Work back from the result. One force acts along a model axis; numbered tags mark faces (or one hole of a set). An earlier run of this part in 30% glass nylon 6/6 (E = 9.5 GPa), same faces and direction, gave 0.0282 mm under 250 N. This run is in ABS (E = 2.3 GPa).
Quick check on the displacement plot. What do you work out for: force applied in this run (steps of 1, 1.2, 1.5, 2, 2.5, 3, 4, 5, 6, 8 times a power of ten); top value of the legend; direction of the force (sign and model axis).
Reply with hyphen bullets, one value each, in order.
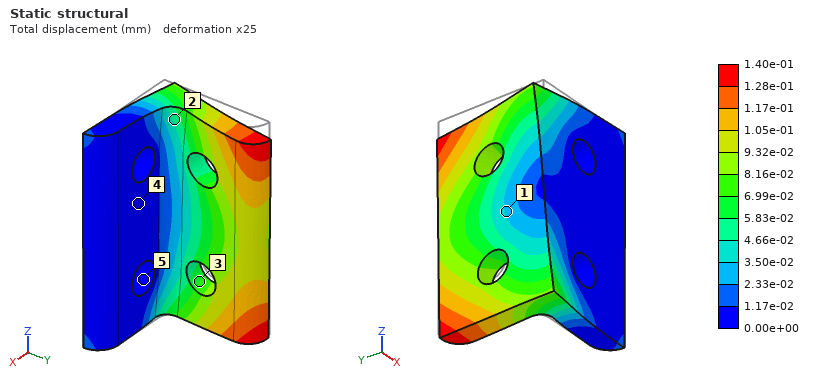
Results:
- 300 N
- 1.40e-01 mm
- -Z
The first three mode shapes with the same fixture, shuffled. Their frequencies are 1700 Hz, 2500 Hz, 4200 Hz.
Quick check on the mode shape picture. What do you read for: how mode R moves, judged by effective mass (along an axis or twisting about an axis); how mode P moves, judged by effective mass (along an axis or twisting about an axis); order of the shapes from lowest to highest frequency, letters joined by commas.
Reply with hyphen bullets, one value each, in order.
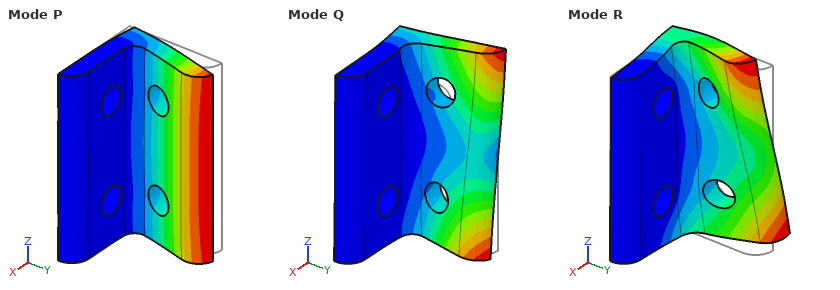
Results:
- along Z
- along X
- P, Q, R
